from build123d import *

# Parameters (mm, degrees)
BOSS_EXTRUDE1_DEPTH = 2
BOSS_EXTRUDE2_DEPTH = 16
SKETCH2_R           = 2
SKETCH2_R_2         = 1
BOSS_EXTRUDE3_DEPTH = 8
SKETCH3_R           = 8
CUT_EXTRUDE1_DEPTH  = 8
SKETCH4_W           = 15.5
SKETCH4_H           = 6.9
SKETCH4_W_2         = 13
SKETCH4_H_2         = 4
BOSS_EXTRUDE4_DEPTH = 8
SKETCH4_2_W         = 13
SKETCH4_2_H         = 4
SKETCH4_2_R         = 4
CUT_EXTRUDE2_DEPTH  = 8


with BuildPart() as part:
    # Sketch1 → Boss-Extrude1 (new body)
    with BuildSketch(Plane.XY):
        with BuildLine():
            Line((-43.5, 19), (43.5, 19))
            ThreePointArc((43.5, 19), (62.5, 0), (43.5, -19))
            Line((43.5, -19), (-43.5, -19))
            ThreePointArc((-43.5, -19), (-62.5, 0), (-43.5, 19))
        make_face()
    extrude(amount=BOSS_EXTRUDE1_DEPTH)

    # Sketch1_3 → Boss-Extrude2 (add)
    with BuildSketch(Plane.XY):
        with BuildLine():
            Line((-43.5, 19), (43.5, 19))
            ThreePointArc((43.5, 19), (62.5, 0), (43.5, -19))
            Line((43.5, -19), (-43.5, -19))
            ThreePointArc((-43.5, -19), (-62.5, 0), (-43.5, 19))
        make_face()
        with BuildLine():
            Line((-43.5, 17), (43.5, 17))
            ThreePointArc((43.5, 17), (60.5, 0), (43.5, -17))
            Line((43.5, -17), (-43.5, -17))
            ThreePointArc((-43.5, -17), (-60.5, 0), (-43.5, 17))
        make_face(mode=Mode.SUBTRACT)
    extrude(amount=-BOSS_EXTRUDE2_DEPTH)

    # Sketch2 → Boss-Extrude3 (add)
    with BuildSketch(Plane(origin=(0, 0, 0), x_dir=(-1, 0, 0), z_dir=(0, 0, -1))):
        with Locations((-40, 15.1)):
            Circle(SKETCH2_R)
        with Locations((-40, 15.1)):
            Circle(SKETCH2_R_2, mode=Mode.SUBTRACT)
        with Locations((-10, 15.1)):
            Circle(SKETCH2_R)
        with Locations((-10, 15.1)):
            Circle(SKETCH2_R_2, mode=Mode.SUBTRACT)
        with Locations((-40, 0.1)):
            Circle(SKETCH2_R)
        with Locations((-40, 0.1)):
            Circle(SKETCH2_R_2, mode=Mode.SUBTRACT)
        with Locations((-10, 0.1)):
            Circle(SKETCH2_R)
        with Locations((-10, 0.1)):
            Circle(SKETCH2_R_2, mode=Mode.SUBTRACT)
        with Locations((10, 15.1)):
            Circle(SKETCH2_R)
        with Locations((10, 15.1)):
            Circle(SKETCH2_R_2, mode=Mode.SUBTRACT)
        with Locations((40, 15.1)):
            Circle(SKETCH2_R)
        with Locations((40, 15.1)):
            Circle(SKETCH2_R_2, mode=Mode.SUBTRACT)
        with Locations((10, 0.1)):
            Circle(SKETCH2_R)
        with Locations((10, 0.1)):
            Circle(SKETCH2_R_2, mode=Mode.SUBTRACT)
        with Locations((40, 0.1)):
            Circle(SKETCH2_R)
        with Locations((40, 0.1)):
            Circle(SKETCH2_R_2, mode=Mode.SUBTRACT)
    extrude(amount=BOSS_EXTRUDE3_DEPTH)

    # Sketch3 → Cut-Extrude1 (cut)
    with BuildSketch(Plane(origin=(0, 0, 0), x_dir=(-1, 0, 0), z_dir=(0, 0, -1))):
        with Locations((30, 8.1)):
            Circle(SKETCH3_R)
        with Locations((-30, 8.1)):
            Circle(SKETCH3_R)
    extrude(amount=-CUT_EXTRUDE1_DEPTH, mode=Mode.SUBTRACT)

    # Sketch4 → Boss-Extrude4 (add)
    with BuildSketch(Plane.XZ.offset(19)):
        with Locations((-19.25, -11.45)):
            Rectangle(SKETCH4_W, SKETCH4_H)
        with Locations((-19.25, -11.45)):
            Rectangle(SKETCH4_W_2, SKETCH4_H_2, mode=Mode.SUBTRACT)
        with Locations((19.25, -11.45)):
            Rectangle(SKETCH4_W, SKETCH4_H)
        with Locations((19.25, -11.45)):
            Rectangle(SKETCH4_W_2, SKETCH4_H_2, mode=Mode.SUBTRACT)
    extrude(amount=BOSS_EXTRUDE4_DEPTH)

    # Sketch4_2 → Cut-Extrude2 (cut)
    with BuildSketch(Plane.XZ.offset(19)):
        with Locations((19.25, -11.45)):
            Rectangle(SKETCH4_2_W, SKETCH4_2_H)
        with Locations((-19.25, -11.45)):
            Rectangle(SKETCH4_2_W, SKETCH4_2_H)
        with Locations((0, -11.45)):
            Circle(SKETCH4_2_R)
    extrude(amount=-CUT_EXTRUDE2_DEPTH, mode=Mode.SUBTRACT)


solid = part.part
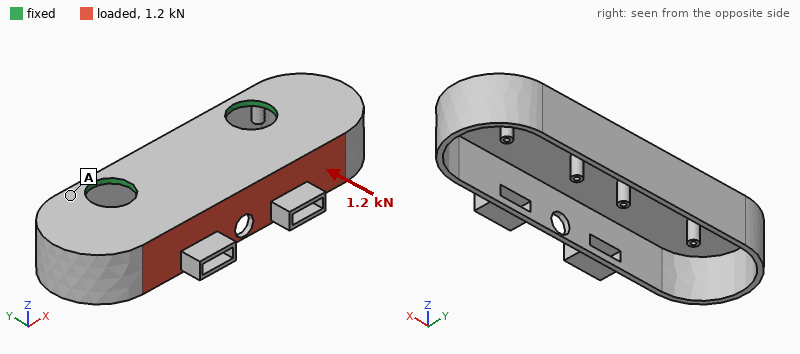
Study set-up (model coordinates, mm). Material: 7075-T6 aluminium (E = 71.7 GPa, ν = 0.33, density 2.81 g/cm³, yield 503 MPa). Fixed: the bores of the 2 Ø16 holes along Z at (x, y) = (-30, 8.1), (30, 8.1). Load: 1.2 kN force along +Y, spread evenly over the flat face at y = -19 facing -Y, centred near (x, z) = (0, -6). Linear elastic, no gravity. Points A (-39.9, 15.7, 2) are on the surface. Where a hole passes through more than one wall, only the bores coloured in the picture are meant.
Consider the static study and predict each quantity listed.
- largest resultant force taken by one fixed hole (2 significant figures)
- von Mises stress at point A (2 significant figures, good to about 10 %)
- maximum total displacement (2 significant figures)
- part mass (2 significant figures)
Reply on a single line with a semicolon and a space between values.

600 N; 14 MPa; 0.61 mm; 52 g
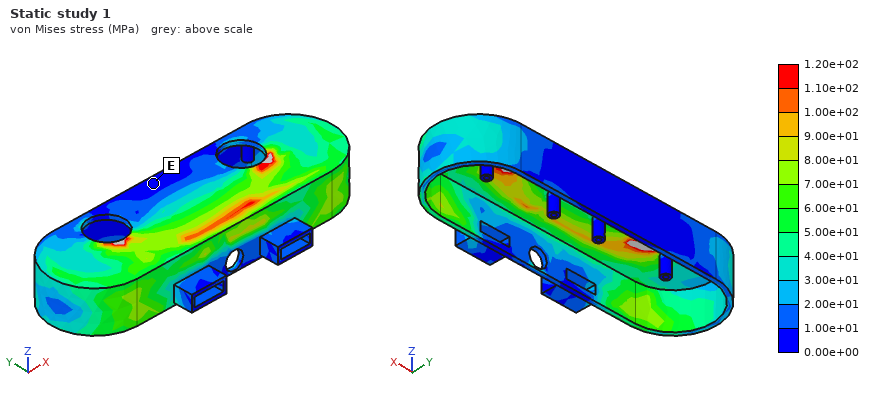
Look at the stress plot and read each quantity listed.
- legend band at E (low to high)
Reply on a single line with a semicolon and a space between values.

0.00e+00 to 1.00e+01 MPa
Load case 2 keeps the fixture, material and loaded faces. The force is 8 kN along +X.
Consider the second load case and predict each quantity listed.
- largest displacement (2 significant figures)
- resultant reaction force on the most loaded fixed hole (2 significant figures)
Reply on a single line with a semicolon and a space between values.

0.87 mm; 4.7 kN
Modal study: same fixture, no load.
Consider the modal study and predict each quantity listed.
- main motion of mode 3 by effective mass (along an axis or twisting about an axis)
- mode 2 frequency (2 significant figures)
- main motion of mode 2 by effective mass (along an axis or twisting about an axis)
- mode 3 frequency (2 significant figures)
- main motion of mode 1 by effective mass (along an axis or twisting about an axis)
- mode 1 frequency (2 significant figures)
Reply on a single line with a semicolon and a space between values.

along Z; 1900 Hz; twisting about Y; 3900 Hz; along Z; 1500 Hz
